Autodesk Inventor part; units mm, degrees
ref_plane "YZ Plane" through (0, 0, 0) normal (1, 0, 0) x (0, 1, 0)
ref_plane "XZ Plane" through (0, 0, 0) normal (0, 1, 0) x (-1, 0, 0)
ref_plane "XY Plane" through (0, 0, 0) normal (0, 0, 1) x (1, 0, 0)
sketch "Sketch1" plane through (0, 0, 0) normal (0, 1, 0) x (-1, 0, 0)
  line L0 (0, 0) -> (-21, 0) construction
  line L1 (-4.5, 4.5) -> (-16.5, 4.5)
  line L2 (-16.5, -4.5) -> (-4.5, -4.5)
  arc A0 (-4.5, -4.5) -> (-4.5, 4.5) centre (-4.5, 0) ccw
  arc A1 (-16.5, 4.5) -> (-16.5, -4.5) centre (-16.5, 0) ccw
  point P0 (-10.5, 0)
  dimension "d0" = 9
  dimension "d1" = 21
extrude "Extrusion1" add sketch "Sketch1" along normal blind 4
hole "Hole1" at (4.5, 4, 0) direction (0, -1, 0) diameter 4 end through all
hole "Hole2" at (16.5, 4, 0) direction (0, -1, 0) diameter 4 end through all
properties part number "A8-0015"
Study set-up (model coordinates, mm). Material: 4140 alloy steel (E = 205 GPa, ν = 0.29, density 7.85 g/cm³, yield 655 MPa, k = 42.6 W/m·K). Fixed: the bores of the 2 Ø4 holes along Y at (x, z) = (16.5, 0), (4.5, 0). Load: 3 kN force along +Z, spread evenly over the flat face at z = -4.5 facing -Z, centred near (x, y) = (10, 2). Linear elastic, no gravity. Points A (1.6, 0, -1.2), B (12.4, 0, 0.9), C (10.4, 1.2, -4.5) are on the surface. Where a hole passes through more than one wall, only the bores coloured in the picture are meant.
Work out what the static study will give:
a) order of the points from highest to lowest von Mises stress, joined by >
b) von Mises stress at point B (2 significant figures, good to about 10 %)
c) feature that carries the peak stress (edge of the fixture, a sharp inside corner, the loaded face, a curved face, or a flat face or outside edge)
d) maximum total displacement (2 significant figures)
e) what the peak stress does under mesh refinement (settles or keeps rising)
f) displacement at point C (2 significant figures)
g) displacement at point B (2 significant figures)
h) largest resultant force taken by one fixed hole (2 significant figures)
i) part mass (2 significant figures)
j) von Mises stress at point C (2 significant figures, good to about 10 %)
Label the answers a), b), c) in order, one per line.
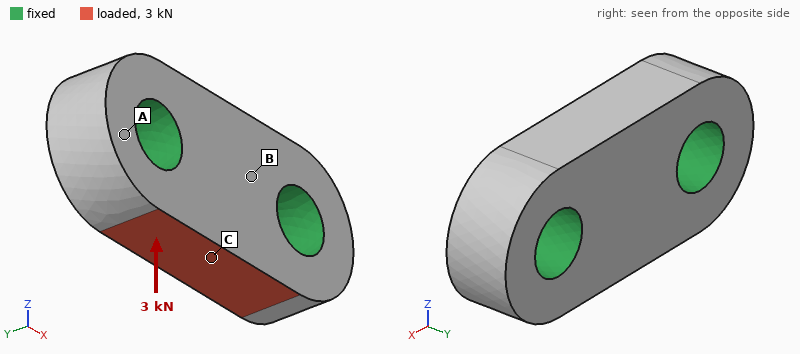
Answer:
a) C > B > A
b) 36 MPa
c) edge of the fixture
d) 2.3 µm
e) keeps rising
f) 2.2 µm
g) 0.99 µm
h) 1.5 kN
i) 4.6 g
j) 64 MPa
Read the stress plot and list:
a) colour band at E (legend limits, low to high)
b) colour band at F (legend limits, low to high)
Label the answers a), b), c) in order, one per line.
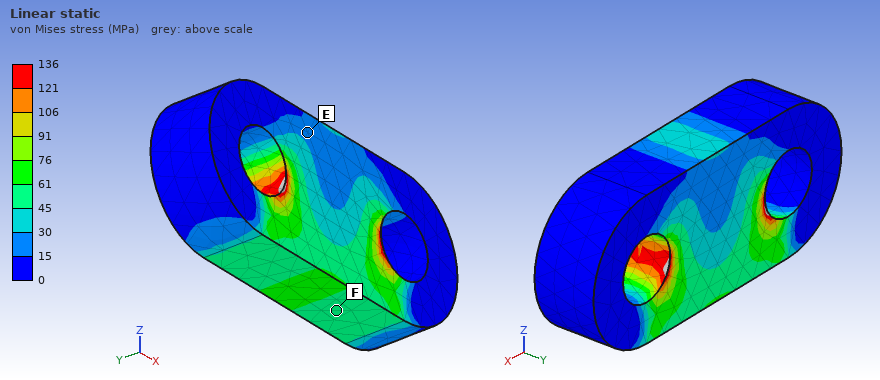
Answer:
a) 15 to 30 MPa
b) 45 to 61 MPa
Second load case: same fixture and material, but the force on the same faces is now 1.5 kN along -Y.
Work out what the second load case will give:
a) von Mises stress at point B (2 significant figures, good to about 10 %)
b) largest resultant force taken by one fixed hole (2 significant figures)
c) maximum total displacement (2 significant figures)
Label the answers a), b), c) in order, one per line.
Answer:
a) 44 MPa
b) 750 N
c) 5.7 µm
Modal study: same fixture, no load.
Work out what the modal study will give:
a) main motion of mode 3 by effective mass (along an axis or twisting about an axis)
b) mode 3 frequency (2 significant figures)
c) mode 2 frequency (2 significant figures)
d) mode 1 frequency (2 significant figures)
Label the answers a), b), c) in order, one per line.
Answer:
a) along Z
b) 140 kHz
c) 120 kHz
d) 120 kHz
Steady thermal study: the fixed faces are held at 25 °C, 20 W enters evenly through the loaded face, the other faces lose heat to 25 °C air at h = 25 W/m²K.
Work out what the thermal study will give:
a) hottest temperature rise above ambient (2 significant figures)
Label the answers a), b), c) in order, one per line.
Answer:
a) 41 K
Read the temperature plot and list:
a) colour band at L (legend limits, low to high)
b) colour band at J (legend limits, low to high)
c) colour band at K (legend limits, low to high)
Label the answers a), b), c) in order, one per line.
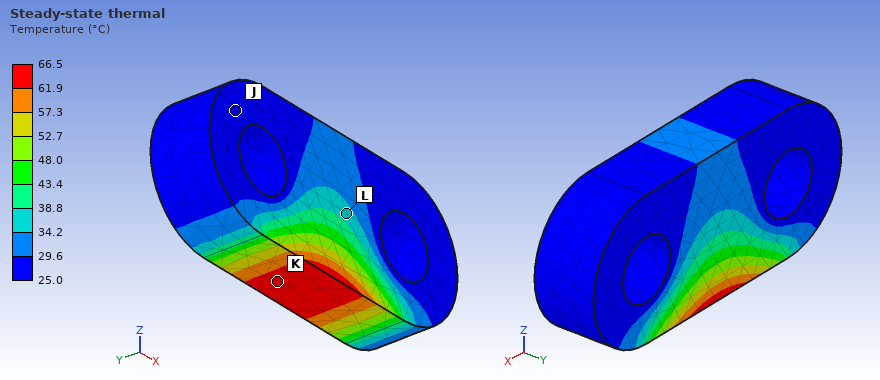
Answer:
a) 34.2 to 38.8 °C
b) 25.0 to 29.6 °C
c) 61.9 to 66.5 °C
